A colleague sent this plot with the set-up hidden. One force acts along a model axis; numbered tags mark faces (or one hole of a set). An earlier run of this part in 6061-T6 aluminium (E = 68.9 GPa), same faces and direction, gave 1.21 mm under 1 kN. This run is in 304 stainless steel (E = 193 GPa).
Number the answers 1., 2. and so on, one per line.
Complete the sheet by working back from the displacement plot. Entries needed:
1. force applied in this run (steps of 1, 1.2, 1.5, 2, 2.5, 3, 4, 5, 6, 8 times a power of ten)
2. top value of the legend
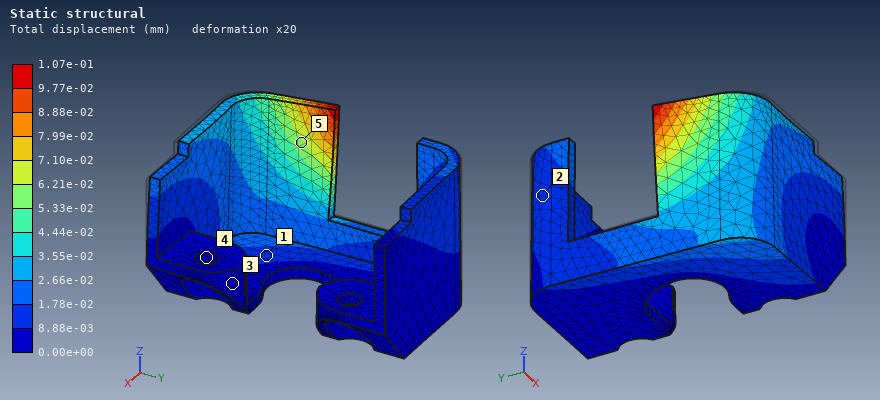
1. 250 N
2. 1.07e-01 mm
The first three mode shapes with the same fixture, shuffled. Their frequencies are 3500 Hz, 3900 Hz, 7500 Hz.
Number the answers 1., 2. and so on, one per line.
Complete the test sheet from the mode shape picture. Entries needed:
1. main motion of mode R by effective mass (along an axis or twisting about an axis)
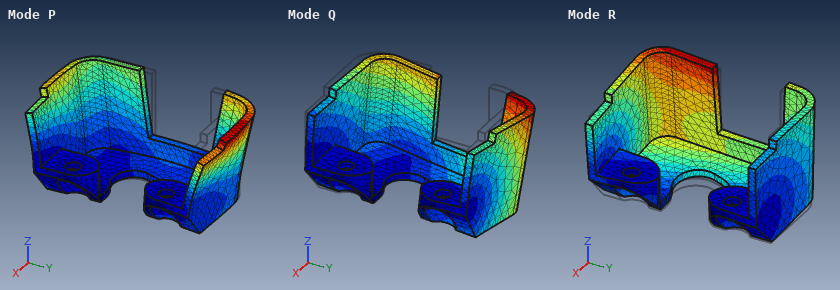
1. along Z
